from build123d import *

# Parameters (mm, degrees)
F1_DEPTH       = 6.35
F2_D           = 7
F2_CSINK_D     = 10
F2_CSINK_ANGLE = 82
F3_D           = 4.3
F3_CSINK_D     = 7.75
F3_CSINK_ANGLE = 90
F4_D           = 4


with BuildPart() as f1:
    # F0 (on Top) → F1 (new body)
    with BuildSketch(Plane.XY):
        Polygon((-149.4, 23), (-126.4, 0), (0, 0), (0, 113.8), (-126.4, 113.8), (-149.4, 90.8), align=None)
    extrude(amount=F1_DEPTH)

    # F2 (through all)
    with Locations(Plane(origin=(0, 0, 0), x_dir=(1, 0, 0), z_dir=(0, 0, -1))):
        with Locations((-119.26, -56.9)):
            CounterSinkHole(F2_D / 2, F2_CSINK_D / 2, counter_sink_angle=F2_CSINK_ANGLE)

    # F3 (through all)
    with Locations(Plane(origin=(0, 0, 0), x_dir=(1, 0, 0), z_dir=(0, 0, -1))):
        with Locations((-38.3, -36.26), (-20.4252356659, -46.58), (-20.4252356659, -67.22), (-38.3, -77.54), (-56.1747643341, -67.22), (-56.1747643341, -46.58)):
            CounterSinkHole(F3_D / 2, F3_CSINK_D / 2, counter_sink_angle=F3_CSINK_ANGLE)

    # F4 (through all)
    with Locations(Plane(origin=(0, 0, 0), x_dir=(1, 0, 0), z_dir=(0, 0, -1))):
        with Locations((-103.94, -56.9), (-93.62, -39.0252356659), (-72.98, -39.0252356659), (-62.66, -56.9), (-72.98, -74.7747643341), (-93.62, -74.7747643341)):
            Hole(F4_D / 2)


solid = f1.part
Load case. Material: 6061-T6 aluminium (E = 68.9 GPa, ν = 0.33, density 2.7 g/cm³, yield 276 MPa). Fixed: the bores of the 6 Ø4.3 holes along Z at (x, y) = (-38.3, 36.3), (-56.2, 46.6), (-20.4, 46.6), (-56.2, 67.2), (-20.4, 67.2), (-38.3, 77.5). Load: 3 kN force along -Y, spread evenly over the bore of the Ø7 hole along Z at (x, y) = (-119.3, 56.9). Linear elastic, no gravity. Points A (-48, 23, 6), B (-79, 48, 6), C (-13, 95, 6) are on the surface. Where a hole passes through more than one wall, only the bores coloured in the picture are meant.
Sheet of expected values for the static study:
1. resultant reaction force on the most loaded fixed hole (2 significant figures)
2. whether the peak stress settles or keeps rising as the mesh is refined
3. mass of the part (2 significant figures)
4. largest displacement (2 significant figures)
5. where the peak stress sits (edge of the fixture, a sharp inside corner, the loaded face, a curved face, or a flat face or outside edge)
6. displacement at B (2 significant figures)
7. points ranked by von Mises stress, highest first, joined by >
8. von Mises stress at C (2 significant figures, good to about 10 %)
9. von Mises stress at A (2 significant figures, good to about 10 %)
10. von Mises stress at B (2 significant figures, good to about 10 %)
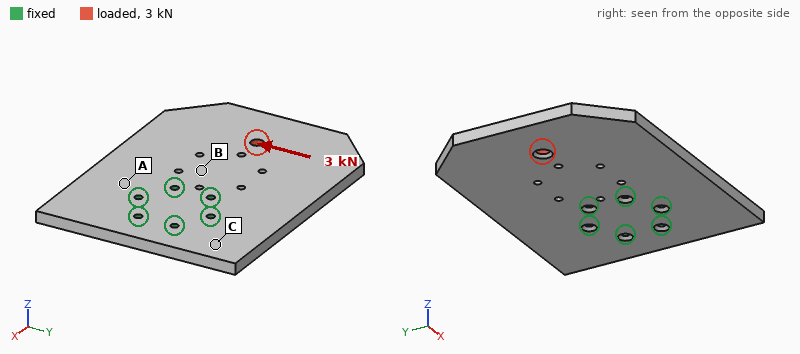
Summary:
2.6 kN
keeps rising
280 g
57 µm
edge of the fixture
15 µm
B > A > C
4.0 MPa
9.2 MPa
15 MPa
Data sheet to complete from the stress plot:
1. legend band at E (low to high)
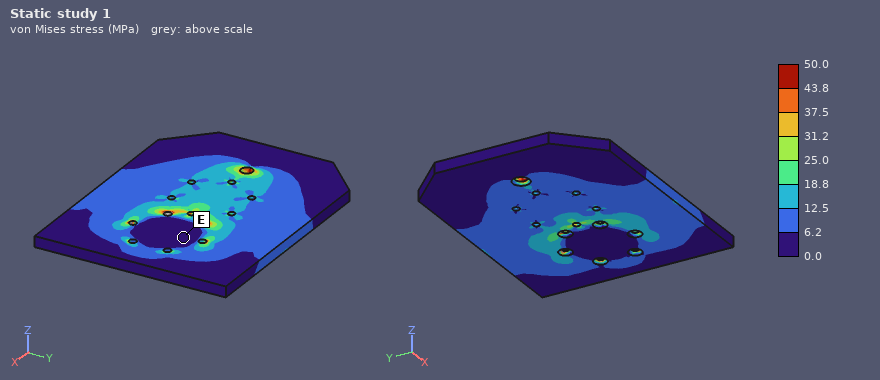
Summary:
0.0 to 6.2 MPa
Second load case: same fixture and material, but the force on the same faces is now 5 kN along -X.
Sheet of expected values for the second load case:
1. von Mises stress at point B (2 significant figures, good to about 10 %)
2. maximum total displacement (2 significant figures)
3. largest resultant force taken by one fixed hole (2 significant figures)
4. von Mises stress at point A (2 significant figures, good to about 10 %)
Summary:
19 MPa
0.11 mm
1.5 kN
6.8 MPa
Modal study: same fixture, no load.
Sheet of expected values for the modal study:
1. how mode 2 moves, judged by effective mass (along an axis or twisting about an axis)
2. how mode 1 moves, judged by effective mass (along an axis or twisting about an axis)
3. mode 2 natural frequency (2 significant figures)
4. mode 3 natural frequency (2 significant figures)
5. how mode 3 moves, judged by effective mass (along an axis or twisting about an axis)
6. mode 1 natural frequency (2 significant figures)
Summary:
twisting about X
along Z
1100 Hz
2300 Hz
along Z
570 Hz
